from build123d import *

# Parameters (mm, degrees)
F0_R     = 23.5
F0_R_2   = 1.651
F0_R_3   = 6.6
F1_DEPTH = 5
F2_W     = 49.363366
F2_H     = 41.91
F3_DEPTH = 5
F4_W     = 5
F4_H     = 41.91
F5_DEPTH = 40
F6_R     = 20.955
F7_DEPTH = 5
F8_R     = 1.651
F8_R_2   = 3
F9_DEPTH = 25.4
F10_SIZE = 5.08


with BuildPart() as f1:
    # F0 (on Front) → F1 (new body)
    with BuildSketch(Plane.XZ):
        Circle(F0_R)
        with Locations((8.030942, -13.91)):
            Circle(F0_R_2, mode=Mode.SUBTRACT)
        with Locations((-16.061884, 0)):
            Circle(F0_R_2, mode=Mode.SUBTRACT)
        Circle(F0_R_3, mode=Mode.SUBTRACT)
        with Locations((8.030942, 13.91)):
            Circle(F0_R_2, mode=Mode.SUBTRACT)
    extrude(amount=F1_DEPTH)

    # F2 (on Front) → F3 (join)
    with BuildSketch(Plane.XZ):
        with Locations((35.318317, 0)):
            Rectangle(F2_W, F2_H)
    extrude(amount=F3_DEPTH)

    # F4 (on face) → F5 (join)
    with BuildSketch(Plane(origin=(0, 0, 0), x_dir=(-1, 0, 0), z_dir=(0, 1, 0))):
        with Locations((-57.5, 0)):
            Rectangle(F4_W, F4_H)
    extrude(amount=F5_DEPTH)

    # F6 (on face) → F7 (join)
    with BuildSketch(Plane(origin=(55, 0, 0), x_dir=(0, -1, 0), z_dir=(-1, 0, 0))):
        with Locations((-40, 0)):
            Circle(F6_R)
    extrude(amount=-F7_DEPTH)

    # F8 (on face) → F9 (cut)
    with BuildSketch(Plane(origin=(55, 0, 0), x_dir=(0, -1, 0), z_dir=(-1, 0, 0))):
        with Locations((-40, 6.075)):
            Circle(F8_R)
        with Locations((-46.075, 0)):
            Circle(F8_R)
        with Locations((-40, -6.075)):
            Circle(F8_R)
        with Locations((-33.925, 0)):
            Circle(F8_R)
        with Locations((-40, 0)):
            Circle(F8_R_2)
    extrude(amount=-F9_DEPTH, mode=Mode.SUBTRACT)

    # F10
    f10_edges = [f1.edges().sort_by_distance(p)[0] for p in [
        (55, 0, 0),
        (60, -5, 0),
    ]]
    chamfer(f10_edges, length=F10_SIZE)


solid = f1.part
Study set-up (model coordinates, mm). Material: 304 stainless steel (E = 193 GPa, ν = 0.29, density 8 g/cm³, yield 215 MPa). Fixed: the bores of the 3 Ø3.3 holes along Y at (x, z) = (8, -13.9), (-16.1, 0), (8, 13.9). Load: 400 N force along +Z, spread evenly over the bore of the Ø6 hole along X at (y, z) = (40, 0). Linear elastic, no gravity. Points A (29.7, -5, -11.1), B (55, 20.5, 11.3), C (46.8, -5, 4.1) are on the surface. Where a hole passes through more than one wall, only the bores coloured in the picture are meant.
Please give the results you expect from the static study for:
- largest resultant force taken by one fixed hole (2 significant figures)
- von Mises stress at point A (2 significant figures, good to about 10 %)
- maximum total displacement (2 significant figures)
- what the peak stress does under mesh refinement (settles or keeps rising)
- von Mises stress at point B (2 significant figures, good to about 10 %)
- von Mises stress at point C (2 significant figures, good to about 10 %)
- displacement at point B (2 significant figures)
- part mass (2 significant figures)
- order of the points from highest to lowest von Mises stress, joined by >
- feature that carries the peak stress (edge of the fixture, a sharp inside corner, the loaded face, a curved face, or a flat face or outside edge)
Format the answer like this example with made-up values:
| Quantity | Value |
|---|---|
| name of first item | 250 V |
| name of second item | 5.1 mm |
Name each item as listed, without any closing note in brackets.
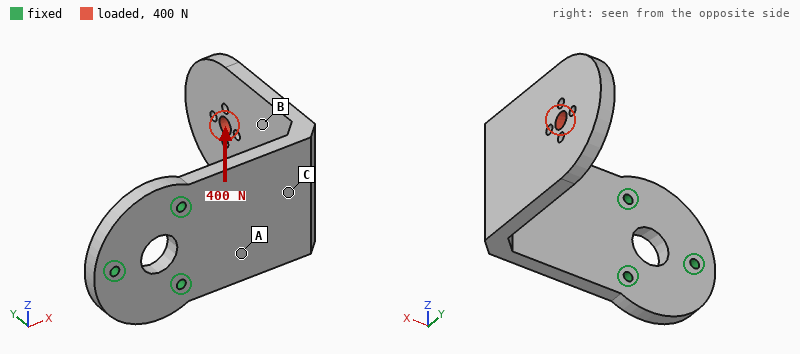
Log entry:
| Quantity | Value |
|---|---|
| largest resultant force taken by one fixed hole | 860 N |
| von Mises stress at point A | 70 MPa |
| maximum total displacement | 0.28 mm |
| what the peak stress does under mesh refinement | keeps rising |
| von Mises stress at point B | 11 MPa |
| von Mises stress at point C | 53 MPa |
| displacement at point B | 0.12 mm |
| part mass | 220 g |
| order of the points from highest to lowest von Mises stress, joined by > | A > C > B |
| feature that carries the peak stress | edge of the fixture |
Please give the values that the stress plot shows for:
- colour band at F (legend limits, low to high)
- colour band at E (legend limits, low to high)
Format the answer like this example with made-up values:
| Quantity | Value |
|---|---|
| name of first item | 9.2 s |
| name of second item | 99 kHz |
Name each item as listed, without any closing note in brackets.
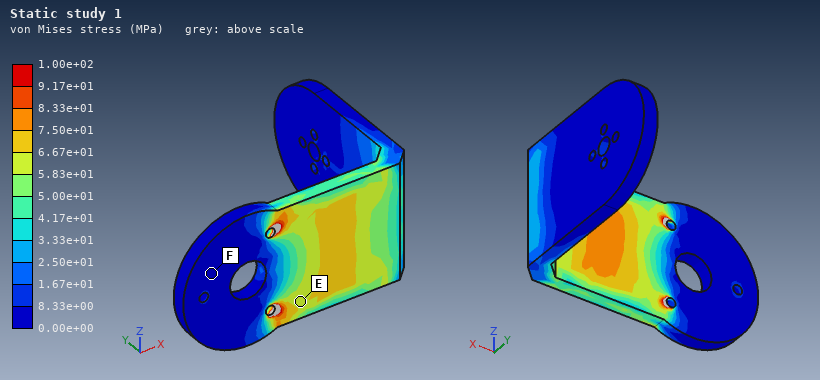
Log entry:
| Quantity | Value |
|---|---|
| colour band at F | 0.00e+00 to 8.33e+00 MPa |
| colour band at E | 5.83e+01 to 6.67e+01 MPa |
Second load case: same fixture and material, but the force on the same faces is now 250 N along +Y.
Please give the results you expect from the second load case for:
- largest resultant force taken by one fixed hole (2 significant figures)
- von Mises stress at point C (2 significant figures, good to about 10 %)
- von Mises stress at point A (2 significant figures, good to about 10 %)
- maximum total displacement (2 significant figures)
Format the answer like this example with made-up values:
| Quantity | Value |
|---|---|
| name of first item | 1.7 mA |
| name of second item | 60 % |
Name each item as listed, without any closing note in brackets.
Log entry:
| Quantity | Value |
|---|---|
| largest resultant force taken by one fixed hole | 180 N |
| von Mises stress at point C | 15 MPa |
| von Mises stress at point A | 38 MPa |
| maximum total displacement | 0.28 mm |
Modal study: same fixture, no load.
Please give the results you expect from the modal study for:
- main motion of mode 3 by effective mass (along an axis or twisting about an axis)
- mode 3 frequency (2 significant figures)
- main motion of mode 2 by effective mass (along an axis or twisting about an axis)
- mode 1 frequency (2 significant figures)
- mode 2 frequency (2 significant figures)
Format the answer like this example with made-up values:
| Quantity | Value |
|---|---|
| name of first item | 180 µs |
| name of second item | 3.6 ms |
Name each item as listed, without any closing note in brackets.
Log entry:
| Quantity | Value |
|---|---|
| main motion of mode 3 by effective mass | along Y |
| mode 3 frequency | 1400 Hz |
| main motion of mode 2 by effective mass | along Z |
| mode 1 frequency | 460 Hz |
| mode 2 frequency | 860 Hz |
